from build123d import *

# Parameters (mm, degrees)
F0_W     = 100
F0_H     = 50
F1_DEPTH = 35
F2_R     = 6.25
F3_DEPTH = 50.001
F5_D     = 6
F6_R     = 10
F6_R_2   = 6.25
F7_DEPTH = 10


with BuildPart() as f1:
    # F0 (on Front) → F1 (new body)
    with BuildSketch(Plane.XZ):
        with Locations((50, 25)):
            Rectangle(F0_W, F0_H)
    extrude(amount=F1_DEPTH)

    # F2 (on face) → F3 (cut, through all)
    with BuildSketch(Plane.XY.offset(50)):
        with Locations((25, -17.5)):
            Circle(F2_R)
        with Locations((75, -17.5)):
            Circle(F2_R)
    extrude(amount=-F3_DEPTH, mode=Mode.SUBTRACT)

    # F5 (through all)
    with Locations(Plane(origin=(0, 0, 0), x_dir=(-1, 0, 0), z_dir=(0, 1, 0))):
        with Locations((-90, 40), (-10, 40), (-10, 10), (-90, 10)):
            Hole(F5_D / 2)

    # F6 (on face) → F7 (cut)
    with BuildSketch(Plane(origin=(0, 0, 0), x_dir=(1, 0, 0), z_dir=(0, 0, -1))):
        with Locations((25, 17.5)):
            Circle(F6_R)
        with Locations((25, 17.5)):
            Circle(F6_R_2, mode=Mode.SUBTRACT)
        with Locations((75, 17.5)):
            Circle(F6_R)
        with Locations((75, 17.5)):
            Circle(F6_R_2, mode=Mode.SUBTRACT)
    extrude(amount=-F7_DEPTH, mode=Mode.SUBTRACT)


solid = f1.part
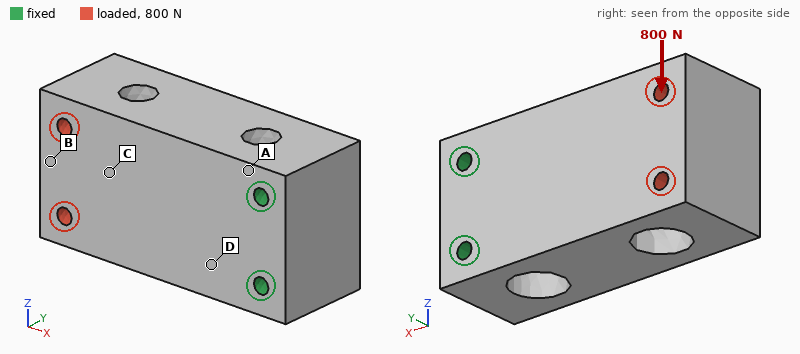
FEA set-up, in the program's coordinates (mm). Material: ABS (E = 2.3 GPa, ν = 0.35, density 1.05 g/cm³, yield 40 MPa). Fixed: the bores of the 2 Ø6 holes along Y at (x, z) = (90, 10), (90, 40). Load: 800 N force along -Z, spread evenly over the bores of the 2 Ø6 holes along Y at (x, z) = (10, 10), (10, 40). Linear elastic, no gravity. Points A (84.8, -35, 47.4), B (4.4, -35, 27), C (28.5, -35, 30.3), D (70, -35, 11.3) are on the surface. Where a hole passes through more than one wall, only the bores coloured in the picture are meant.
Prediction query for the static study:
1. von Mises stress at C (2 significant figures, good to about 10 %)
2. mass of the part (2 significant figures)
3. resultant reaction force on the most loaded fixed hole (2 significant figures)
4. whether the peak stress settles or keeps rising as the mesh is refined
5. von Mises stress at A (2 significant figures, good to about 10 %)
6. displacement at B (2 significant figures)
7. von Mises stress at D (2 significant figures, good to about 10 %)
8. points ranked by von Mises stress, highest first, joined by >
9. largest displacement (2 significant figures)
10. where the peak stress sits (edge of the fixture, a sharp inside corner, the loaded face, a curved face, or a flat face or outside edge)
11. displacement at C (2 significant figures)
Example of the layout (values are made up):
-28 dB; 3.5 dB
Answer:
1.5 MPa; 160 g; 2.0 kN; keeps rising; 3.8 MPa; 0.34 mm; 3.1 MPa; A > D > C > B; 0.39 mm; edge of the fixture; 0.22 mm
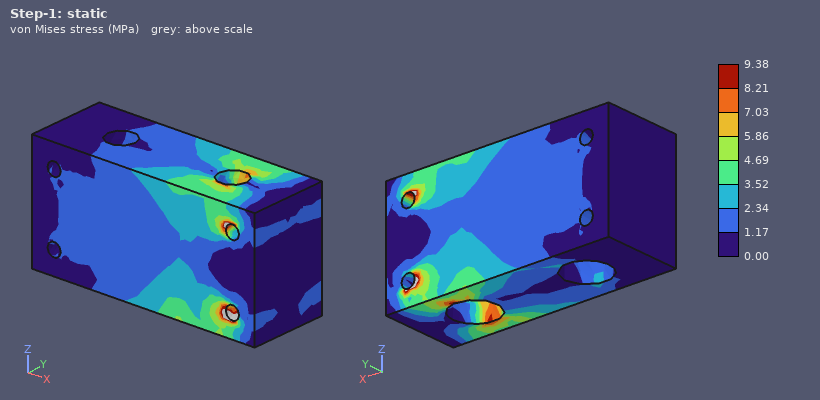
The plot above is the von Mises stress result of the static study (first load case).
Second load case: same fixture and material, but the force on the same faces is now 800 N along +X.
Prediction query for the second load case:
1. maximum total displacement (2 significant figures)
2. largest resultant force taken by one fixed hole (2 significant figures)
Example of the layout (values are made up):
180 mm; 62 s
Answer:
31 µm; 410 N
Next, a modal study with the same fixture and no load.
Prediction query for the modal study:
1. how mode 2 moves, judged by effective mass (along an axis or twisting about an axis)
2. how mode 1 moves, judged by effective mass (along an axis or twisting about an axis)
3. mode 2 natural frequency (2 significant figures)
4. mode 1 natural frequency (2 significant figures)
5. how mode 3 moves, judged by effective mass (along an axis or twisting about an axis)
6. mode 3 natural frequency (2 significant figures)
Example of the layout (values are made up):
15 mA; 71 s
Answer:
along Z; along Y; 1100 Hz; 880 Hz; twisting about X; 2000 Hz
